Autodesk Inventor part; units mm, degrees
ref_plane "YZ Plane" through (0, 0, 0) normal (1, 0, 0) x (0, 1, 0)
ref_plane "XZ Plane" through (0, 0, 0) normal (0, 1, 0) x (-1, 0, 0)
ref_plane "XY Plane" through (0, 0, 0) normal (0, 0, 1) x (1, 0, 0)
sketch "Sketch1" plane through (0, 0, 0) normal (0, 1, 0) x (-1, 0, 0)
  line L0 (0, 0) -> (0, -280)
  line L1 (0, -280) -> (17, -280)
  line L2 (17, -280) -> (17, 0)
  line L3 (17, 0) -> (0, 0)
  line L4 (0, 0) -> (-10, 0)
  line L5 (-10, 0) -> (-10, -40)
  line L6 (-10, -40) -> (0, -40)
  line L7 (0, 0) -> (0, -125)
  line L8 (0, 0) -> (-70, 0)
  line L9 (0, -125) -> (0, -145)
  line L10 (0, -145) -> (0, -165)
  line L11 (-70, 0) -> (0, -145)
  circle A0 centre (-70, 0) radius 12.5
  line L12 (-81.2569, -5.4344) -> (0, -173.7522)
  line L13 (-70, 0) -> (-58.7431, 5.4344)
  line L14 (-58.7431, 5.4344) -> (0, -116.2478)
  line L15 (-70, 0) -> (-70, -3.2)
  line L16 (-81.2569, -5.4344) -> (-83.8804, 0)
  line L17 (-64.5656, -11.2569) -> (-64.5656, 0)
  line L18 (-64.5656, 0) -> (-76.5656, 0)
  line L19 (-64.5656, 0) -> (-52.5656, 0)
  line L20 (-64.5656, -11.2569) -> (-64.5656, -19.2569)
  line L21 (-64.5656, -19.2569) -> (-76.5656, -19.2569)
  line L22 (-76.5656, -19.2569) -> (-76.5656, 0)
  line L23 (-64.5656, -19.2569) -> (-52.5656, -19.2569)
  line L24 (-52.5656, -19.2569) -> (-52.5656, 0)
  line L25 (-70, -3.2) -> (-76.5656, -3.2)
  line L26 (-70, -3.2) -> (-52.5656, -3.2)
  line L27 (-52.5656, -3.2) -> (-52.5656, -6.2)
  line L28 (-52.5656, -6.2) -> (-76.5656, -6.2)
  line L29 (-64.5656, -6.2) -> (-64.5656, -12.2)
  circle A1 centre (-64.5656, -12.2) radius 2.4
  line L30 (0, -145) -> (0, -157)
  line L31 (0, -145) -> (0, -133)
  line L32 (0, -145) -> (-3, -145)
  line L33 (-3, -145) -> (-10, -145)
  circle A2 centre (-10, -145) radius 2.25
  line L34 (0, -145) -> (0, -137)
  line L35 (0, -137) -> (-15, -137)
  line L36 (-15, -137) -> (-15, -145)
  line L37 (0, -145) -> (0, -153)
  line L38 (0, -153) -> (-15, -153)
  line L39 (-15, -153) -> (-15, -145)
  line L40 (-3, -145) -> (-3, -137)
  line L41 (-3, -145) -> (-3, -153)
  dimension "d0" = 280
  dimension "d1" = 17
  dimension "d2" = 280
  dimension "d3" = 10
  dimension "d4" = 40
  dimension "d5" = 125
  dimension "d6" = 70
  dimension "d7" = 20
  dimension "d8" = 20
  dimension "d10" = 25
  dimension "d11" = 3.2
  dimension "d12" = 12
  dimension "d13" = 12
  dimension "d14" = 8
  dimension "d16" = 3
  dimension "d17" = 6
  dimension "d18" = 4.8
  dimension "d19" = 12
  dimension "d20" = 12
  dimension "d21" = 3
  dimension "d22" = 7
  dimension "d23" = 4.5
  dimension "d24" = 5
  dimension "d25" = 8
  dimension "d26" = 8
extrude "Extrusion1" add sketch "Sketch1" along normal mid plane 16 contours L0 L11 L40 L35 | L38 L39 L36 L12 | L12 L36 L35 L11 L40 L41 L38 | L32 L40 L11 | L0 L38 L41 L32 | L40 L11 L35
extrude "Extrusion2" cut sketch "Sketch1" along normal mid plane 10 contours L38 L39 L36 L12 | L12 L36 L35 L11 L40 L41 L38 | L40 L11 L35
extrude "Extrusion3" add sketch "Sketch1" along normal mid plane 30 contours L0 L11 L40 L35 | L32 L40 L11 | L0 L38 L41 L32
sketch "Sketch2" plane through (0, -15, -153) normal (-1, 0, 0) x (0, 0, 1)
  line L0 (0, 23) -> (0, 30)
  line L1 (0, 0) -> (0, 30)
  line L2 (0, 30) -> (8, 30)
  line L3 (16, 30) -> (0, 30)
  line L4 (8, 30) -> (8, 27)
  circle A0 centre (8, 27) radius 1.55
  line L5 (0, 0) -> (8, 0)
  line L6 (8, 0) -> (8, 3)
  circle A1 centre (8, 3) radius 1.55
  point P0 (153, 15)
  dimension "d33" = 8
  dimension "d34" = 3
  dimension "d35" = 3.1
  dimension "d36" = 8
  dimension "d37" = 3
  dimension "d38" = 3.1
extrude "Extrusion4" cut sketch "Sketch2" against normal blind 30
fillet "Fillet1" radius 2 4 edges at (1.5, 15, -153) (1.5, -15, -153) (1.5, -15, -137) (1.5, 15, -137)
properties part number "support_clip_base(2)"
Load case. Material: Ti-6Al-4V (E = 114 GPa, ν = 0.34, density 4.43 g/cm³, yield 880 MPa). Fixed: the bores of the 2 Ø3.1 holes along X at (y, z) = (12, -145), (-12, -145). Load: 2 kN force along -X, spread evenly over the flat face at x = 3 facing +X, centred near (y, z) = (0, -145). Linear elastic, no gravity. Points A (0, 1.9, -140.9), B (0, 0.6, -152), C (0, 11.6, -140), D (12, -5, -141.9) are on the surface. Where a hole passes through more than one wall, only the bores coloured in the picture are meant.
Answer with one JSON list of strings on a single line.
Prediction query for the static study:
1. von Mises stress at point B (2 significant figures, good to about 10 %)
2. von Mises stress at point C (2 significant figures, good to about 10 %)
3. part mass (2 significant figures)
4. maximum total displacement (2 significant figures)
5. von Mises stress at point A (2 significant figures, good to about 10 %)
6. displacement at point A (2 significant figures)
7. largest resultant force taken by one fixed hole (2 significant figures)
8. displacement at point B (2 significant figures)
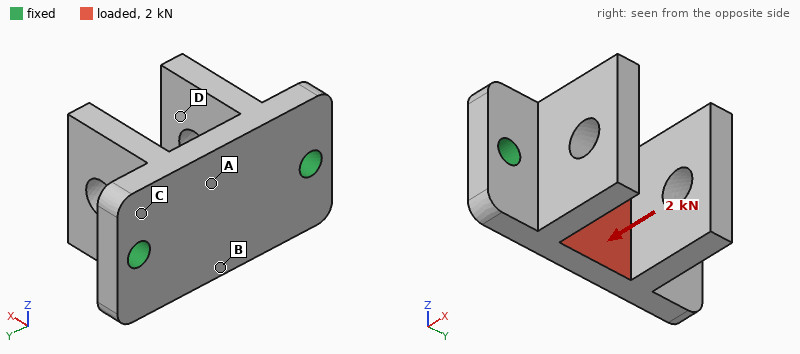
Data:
["160 MPa", "65 MPa", "11 g", "62 µm", "140 MPa", "34 µm", "1.0 kN", "38 µm"]
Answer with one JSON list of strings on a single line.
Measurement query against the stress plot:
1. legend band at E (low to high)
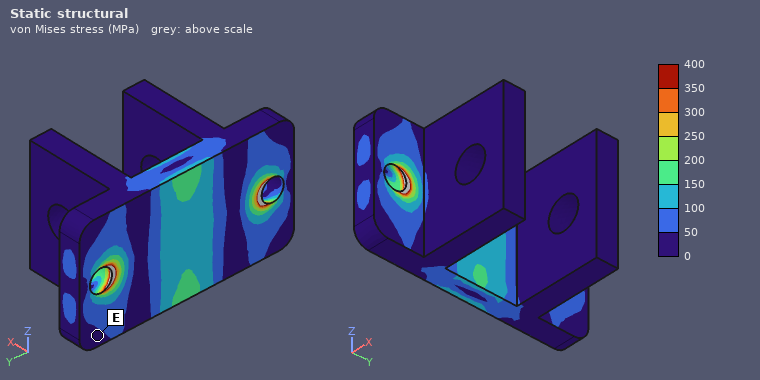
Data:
["0 to 50 MPa"]
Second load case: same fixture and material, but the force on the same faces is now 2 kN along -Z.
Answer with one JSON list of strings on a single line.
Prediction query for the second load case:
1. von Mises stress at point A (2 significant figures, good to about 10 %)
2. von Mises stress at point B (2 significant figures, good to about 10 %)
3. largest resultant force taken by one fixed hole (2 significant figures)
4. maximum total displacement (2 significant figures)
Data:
["37 MPa", "78 MPa", "1.0 kN", "23 µm"]
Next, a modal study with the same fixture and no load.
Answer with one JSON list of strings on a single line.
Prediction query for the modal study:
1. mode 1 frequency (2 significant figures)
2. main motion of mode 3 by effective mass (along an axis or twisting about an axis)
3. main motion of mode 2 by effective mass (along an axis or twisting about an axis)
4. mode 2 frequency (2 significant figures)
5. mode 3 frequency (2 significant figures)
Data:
["10 kHz", "along Y", "along Z", "11 kHz", "13 kHz"]
